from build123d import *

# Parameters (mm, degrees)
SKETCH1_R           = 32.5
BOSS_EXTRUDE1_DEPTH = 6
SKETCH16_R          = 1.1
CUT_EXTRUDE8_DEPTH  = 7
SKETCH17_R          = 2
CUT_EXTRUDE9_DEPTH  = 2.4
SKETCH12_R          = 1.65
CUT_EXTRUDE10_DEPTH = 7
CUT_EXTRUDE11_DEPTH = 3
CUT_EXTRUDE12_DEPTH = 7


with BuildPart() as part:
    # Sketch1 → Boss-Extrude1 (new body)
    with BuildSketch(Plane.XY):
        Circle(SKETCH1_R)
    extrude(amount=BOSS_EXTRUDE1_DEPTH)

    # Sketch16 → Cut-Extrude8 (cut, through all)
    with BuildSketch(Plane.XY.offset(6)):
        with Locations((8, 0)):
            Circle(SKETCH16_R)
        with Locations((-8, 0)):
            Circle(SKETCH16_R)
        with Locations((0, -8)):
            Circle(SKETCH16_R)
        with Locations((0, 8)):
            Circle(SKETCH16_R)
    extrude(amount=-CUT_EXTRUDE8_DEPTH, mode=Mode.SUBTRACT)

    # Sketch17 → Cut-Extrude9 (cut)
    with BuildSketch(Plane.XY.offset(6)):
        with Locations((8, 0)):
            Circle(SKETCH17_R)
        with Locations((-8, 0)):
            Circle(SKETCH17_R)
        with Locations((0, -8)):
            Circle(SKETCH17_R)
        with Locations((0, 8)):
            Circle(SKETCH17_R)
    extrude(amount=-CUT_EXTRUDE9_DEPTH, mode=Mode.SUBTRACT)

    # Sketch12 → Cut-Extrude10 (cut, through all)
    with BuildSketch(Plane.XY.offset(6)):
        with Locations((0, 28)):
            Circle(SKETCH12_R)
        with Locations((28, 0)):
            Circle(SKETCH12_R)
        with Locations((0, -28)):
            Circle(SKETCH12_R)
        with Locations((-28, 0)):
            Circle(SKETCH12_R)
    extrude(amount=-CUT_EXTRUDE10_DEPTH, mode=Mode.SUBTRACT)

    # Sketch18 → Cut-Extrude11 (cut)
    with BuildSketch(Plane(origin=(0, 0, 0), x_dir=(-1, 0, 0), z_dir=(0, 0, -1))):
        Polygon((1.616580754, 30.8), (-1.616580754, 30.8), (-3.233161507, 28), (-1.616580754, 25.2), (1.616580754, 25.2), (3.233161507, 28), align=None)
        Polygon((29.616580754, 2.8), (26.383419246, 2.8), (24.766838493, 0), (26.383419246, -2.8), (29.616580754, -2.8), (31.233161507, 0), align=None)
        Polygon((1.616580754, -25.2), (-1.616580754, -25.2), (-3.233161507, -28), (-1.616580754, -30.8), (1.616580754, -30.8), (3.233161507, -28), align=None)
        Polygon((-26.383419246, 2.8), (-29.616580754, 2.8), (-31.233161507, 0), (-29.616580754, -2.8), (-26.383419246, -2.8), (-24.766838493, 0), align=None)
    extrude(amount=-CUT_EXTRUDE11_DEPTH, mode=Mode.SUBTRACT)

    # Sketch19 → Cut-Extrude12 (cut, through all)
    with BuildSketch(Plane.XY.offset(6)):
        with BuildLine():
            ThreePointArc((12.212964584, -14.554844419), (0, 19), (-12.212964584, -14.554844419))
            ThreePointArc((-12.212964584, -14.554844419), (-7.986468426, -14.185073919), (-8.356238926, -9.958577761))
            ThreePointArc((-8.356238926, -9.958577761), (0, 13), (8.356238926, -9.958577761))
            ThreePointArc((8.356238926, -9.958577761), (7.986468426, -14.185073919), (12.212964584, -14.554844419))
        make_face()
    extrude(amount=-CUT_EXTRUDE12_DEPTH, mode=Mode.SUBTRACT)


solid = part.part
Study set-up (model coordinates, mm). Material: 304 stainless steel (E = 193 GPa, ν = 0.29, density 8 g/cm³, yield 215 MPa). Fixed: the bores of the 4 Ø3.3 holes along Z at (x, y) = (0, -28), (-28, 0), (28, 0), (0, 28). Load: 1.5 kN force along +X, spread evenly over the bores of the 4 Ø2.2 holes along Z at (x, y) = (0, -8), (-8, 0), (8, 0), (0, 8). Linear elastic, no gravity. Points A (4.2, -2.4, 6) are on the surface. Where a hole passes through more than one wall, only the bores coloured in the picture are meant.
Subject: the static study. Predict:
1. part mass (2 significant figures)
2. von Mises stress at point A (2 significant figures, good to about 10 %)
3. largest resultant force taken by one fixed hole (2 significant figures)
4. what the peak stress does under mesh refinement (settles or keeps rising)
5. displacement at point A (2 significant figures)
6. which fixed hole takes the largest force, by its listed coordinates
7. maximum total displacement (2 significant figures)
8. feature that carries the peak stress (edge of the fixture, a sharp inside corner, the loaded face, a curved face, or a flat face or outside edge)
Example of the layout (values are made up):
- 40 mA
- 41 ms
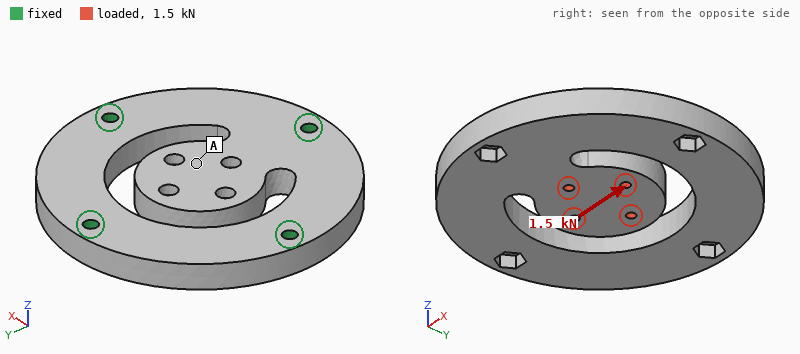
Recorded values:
- 130 g
- 18 MPa
- 1.4 kN
- keeps rising
- 20 µm
- (0, -28)
- 42 µm
- edge of the fixture
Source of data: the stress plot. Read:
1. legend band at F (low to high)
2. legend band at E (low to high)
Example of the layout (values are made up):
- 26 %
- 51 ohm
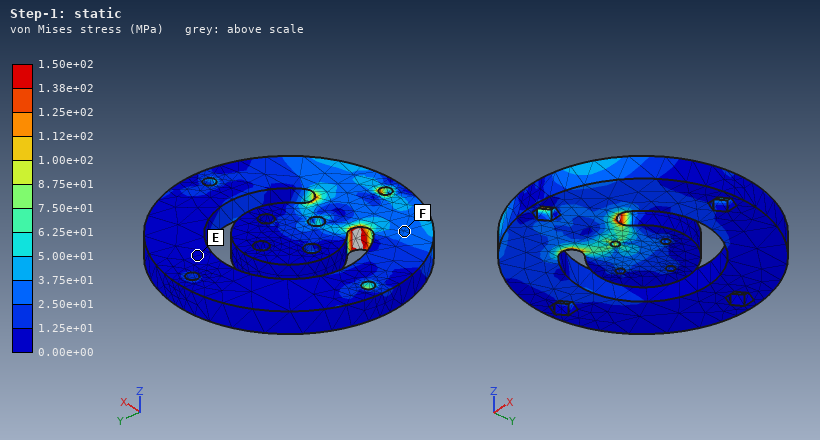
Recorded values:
- 2.50e+01 to 3.75e+01 MPa
- 0.00e+00 to 1.25e+01 MPa
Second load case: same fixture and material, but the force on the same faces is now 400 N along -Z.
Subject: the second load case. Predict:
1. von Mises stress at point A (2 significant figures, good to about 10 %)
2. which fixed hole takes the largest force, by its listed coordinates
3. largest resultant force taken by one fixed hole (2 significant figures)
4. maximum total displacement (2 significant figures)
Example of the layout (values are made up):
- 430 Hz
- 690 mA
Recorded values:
- 16 MPa
- (0, -28)
- 370 N
- 81 µm
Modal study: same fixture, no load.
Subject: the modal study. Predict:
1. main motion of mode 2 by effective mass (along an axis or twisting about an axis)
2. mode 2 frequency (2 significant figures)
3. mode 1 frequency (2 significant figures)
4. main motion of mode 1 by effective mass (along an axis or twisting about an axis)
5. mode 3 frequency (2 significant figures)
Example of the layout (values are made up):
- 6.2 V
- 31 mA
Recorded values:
- along X
- 7000 Hz
- 2800 Hz
- along Z
- 8300 Hz
